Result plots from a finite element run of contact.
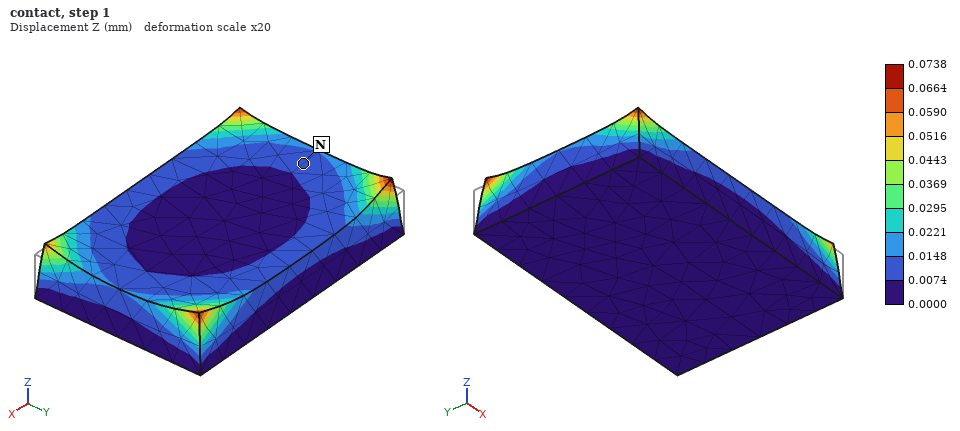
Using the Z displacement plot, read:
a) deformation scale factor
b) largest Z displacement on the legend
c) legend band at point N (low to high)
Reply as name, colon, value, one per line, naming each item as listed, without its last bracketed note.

deformation scale factor: 20
largest Z displacement on the legend: 0.0738 mm
legend band at point N: 0.0074 to 0.0148 mm
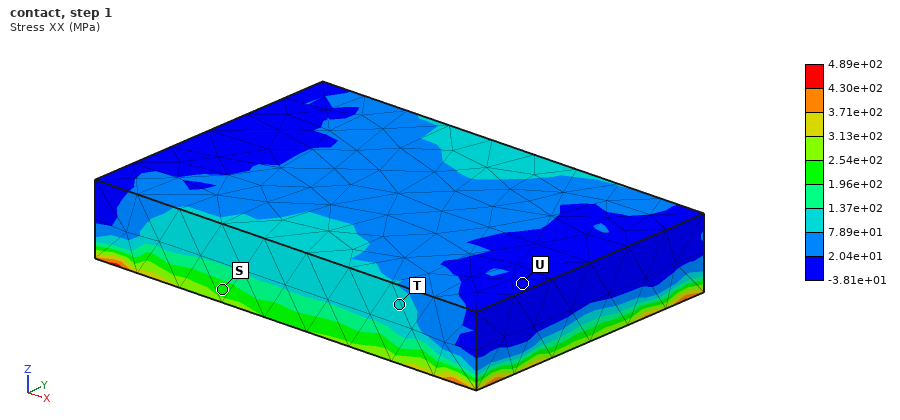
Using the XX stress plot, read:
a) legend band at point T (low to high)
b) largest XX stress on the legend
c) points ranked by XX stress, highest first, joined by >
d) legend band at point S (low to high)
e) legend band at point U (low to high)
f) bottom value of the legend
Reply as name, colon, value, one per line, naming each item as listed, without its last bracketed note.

legend band at point T: 7.89e+01 to 1.37e+02 MPa
largest XX stress on the legend: 4.89e+02 MPa
points ranked by XX stress, highest first, joined by >: S > T > U
legend band at point S: 1.96e+02 to 2.54e+02 MPa
legend band at point U: -3.81e+01 to 2.04e+01 MPa
bottom value of the legend: -3.81e+01 MPa
